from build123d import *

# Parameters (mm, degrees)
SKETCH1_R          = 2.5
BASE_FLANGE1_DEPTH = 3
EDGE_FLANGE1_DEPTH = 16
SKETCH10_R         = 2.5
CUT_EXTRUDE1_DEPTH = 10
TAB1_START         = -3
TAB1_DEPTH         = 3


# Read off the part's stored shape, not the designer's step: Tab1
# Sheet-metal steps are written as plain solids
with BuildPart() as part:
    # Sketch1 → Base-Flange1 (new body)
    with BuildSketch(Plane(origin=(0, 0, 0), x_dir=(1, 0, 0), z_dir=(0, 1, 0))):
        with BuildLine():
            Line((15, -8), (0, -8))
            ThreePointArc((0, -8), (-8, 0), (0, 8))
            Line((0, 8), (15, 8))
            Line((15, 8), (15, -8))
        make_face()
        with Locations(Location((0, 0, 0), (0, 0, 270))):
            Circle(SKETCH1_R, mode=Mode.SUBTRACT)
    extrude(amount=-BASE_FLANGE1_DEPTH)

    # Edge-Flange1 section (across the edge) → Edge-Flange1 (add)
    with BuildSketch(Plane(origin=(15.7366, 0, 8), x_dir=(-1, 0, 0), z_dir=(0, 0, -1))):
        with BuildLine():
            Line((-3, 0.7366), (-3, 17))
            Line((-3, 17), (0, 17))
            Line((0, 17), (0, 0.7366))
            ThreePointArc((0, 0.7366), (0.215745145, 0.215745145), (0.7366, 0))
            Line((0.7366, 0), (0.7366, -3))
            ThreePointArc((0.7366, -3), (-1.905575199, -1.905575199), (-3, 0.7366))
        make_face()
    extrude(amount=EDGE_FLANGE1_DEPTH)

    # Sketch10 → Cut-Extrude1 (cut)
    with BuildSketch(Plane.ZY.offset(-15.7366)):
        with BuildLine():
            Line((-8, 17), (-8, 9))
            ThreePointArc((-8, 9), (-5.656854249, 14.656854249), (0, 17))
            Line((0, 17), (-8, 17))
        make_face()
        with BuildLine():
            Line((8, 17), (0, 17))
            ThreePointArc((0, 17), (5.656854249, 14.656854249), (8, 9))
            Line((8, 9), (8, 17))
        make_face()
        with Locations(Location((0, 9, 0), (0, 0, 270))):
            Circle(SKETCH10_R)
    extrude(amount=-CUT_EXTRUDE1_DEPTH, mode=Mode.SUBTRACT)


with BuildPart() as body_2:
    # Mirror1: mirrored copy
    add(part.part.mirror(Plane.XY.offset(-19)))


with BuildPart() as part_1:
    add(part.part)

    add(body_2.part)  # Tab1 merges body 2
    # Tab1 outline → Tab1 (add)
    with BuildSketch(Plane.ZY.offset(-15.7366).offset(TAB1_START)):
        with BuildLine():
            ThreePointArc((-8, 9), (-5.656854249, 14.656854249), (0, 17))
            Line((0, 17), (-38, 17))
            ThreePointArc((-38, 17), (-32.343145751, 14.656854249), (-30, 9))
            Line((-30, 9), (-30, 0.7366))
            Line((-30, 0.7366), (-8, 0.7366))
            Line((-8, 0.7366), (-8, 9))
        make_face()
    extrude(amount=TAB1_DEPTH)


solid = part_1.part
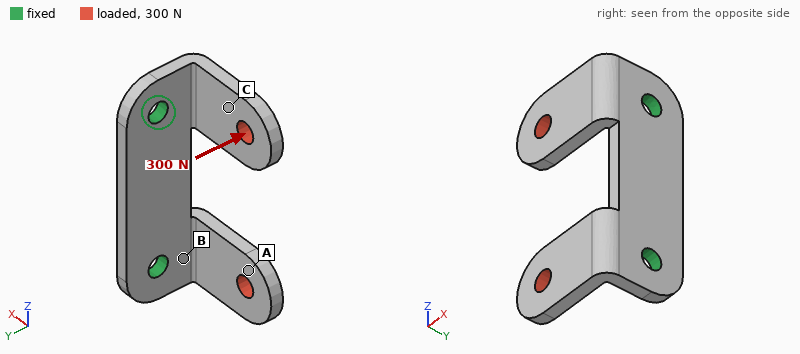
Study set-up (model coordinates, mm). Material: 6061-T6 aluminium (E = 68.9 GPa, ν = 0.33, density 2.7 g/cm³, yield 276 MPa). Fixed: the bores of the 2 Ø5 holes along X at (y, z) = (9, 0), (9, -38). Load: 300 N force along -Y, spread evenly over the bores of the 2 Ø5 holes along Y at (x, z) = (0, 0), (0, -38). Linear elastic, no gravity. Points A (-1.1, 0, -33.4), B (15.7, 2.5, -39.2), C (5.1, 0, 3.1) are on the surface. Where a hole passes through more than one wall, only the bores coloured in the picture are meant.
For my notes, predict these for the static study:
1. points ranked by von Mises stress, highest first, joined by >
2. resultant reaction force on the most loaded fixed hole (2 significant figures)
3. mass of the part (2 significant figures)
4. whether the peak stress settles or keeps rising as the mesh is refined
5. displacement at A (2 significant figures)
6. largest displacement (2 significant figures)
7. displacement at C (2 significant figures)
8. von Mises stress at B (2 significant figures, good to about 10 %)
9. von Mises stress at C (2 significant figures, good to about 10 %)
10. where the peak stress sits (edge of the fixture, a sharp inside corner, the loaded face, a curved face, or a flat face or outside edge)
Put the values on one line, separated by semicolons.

B > C > A; 150 N; 13 g; keeps rising; 0.25 mm; 0.37 mm; 0.15 mm; 100 MPa; 34 MPa; a sharp inside corner
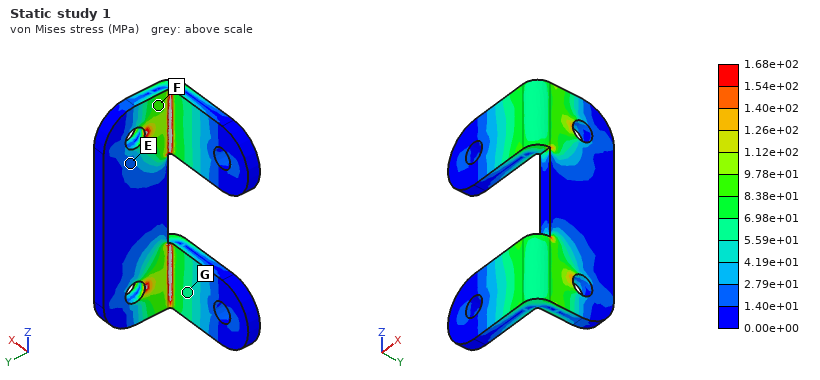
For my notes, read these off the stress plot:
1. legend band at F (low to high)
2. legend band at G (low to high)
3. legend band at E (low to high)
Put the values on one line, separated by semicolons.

8.38e+01 to 9.78e+01 MPa; 5.59e+01 to 6.98e+01 MPa; 1.40e+01 to 2.79e+01 MPa
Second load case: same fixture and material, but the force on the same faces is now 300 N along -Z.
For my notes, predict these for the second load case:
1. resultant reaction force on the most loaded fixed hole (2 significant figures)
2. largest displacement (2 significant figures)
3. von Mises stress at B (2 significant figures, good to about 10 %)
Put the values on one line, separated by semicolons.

170 N; 0.10 mm; 57 MPa
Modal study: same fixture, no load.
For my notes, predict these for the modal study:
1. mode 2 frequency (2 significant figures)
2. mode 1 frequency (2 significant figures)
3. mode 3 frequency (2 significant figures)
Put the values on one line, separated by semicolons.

3000 Hz; 3000 Hz; 4700 Hz
